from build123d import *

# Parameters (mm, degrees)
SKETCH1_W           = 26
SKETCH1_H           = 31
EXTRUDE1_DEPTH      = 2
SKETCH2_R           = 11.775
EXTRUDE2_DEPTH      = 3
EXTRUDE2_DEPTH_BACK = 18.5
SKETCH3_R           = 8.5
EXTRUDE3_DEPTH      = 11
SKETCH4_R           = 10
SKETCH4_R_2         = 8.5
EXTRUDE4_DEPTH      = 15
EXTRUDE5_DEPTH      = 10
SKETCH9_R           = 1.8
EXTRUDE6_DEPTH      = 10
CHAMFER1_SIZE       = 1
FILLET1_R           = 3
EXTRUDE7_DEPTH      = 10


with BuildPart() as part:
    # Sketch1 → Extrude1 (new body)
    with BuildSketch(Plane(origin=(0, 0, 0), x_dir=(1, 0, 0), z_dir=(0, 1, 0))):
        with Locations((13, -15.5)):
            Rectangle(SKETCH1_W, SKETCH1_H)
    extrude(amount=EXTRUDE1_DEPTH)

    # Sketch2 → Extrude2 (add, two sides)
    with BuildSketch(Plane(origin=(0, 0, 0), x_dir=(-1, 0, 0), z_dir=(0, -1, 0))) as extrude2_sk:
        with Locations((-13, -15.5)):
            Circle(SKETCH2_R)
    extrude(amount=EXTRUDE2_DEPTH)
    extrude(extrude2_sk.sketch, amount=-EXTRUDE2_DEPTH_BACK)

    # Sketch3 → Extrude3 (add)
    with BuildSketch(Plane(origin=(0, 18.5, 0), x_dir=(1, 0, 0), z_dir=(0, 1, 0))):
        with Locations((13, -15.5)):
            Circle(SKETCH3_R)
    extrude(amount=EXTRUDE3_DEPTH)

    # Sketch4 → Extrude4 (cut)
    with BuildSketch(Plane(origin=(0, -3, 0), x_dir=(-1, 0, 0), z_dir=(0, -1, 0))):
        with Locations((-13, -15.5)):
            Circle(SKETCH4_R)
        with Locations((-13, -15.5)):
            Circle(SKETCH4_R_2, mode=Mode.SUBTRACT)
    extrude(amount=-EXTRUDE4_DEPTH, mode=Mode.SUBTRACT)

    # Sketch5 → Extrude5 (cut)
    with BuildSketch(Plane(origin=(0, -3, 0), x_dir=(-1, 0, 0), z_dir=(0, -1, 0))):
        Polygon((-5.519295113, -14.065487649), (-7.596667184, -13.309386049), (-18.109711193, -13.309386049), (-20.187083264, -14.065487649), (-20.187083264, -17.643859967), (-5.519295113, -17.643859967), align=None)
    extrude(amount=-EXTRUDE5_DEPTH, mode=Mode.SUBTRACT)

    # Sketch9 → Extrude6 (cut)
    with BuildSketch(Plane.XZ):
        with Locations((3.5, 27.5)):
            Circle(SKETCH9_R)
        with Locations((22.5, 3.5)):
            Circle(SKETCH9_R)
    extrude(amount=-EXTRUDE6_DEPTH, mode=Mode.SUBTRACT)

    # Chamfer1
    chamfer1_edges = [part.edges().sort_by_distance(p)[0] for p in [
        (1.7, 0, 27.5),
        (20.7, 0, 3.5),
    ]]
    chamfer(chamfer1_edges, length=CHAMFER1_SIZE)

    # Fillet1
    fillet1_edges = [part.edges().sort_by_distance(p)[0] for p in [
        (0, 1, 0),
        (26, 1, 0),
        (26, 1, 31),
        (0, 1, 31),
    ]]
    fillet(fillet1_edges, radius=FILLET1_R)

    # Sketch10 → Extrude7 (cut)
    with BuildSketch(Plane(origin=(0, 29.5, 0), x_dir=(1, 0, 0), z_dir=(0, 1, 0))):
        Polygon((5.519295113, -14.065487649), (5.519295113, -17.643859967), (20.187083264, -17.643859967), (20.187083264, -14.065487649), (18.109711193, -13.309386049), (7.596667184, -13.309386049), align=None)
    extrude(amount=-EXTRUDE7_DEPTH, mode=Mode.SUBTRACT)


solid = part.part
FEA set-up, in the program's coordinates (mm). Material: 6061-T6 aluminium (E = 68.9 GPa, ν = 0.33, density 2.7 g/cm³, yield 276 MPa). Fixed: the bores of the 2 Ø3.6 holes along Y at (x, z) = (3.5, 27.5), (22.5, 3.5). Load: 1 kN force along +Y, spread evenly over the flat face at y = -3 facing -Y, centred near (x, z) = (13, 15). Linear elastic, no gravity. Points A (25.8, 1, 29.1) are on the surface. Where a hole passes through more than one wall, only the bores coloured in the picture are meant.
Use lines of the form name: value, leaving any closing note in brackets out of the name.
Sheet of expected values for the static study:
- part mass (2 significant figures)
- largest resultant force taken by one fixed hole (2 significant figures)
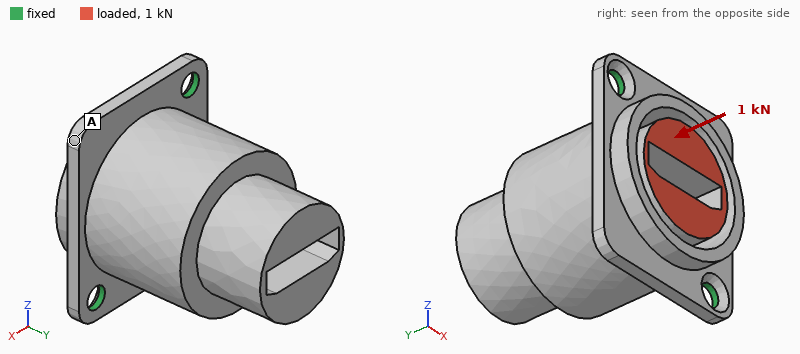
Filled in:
part mass: 27 g
largest resultant force taken by one fixed hole: 510 N
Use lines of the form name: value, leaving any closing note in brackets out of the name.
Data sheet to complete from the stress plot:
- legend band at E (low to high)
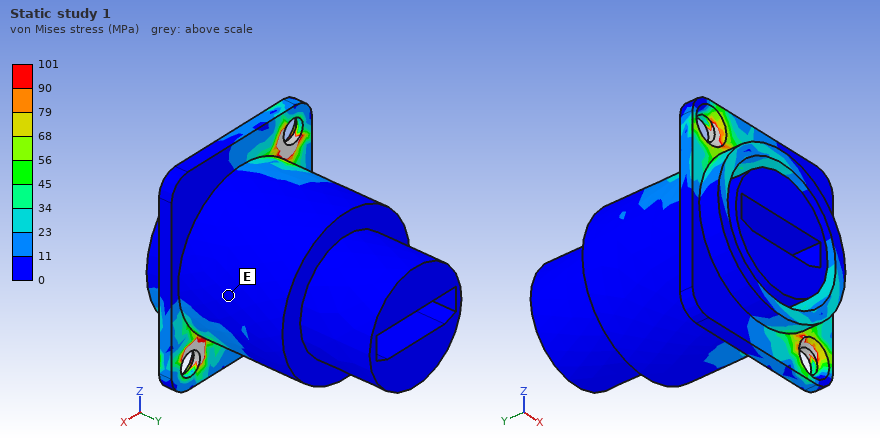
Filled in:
legend band at E: 0 to 11 MPa
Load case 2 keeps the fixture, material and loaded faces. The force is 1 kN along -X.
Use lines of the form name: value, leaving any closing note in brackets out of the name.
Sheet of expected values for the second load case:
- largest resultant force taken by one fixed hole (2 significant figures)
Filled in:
largest resultant force taken by one fixed hole: 510 N
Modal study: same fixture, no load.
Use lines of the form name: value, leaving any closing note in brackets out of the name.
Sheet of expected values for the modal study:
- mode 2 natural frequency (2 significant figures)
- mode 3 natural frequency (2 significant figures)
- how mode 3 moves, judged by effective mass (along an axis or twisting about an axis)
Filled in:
mode 2 natural frequency: 5800 Hz
mode 3 natural frequency: 7100 Hz
how mode 3 moves, judged by effective mass: along Y
